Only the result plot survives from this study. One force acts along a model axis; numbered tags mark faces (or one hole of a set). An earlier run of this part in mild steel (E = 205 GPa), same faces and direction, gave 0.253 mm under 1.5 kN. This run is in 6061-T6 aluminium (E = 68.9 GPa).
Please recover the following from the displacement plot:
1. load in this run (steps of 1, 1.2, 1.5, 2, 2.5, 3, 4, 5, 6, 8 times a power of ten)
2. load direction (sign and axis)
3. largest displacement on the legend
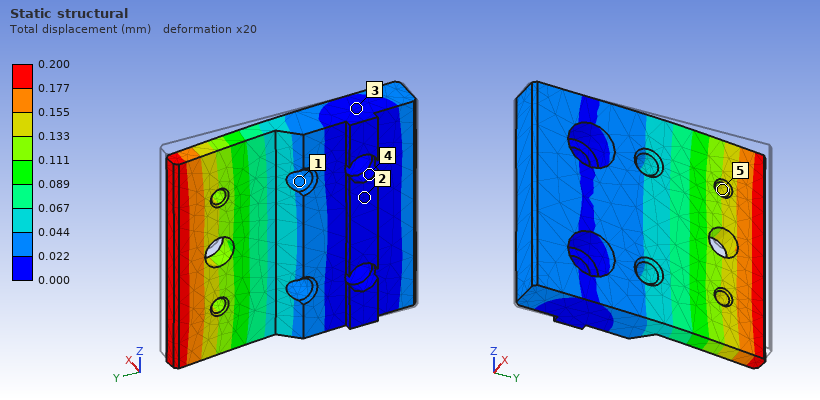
400 N
-X
0.200 mm
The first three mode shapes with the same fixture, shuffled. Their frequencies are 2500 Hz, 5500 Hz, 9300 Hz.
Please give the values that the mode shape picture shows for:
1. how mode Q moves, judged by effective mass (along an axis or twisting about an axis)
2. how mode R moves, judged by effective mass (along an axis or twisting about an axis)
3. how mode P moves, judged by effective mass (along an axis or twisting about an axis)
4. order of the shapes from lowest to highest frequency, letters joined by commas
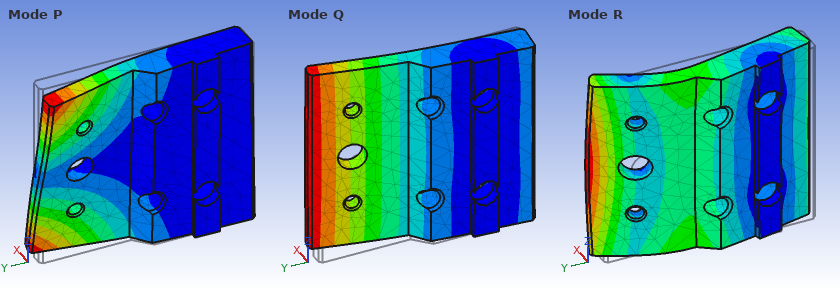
along X
along Y
twisting about Y
Q, P, R
